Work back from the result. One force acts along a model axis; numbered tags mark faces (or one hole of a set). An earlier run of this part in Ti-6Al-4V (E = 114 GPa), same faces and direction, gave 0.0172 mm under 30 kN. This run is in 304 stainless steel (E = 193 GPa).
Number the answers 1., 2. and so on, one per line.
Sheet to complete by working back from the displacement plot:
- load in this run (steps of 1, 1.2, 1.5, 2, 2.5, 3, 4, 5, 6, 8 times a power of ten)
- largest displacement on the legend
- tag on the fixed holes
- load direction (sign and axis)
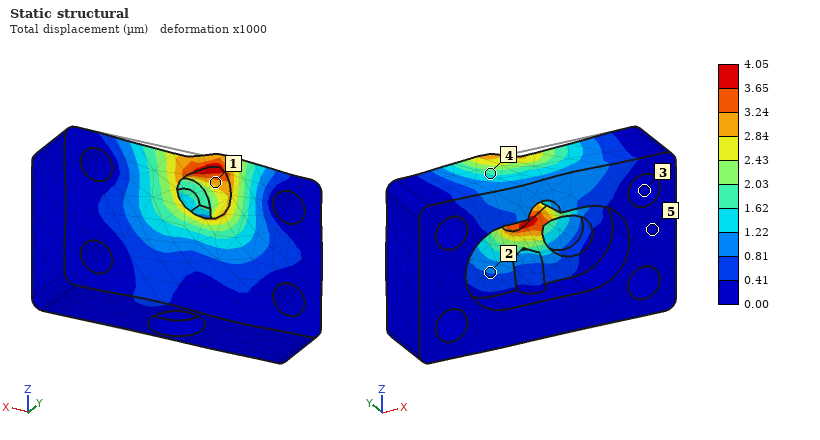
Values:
1. 12 kN
2. 4.05 µm
3. 3
4. -X
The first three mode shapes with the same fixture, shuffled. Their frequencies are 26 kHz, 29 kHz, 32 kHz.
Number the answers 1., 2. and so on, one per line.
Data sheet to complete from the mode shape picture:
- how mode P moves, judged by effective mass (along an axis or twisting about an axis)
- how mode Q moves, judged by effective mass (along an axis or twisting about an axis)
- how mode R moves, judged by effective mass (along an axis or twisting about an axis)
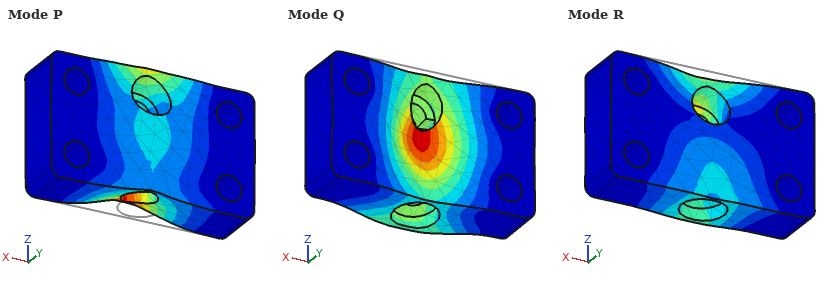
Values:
1. along Z
2. along Y
3. along Z
